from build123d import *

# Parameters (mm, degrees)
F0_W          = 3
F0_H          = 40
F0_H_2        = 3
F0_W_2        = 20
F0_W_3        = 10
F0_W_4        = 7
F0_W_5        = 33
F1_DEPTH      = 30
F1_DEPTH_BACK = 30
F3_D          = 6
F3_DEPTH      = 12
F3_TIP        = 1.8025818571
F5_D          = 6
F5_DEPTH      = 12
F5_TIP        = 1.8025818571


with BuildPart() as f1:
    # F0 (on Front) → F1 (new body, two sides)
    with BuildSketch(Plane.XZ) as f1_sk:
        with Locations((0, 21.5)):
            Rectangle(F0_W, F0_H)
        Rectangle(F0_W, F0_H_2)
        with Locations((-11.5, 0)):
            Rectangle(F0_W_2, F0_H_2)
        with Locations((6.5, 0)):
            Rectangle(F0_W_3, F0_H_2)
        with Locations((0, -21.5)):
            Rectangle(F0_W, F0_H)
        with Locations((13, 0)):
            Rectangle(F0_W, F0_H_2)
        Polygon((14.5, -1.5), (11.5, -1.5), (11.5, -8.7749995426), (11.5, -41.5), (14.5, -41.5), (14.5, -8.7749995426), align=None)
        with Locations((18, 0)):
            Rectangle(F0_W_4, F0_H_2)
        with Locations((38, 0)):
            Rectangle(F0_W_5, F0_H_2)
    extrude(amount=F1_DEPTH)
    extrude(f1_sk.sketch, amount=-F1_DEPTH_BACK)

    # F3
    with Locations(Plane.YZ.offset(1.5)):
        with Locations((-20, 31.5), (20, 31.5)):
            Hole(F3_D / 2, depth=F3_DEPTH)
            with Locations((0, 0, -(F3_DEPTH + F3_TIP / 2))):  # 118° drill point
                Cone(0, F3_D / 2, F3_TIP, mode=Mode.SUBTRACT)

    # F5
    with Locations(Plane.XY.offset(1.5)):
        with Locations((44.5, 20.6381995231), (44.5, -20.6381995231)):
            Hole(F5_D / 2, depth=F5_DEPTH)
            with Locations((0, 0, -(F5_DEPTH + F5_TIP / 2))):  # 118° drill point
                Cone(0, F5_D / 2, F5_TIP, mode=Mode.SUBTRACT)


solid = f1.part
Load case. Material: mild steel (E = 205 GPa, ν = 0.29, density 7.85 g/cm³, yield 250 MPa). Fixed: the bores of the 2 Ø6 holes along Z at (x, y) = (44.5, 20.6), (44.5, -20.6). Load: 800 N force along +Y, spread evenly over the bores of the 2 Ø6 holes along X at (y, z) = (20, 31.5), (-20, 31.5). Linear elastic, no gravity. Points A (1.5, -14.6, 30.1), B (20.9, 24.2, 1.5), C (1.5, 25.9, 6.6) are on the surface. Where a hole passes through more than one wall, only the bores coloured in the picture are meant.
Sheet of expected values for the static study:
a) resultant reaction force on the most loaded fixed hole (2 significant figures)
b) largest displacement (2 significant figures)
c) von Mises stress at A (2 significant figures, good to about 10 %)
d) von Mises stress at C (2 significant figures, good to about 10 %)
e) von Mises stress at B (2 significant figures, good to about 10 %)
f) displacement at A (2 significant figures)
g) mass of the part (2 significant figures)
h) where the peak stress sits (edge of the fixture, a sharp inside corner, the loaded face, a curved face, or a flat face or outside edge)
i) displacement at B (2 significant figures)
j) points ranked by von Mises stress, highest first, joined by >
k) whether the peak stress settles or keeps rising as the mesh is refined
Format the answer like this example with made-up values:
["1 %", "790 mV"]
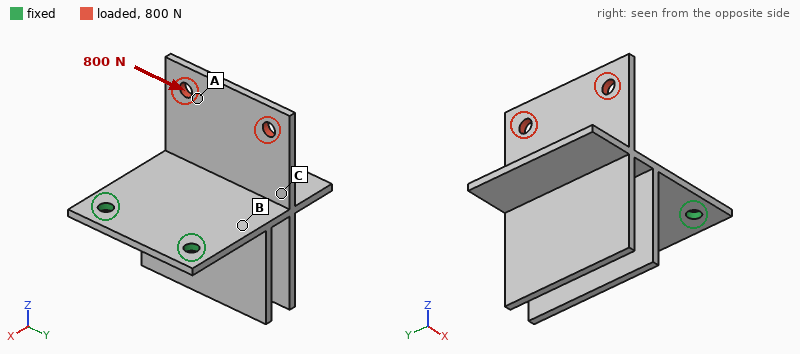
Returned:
["1.1 kN", "0.51 mm", "17 MPa", "58 MPa", "130 MPa", "0.34 mm", "270 g", "edge of the fixture", "0.13 mm", "B > C > A", "keeps rising"]
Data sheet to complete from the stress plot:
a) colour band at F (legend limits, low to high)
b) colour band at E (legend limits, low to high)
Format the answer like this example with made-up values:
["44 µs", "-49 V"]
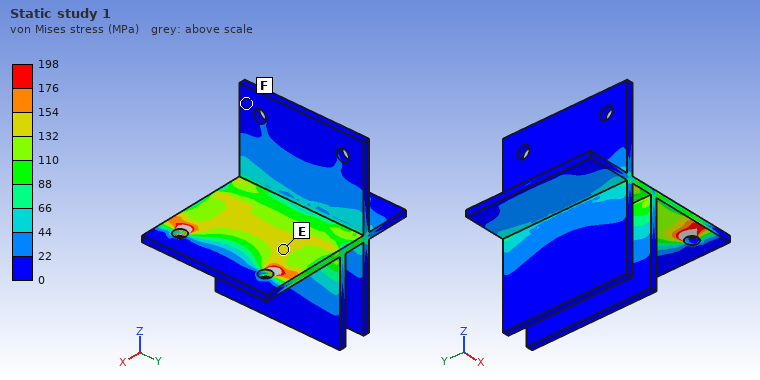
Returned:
["0 to 22 MPa", "132 to 154 MPa"]
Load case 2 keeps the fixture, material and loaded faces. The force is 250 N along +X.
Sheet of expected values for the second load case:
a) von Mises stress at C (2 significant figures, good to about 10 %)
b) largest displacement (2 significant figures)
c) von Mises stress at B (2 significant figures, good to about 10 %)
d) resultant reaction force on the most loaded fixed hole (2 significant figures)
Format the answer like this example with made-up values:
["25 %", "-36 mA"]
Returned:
["65 MPa", "0.67 mm", "82 MPa", "130 N"]
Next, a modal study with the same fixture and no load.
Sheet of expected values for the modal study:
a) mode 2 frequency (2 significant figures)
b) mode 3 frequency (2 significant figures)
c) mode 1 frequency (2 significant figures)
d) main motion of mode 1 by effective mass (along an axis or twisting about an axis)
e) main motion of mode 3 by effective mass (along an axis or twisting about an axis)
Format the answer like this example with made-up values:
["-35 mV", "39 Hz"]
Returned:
["670 Hz", "990 Hz", "280 Hz", "along Z", "along Z"]
